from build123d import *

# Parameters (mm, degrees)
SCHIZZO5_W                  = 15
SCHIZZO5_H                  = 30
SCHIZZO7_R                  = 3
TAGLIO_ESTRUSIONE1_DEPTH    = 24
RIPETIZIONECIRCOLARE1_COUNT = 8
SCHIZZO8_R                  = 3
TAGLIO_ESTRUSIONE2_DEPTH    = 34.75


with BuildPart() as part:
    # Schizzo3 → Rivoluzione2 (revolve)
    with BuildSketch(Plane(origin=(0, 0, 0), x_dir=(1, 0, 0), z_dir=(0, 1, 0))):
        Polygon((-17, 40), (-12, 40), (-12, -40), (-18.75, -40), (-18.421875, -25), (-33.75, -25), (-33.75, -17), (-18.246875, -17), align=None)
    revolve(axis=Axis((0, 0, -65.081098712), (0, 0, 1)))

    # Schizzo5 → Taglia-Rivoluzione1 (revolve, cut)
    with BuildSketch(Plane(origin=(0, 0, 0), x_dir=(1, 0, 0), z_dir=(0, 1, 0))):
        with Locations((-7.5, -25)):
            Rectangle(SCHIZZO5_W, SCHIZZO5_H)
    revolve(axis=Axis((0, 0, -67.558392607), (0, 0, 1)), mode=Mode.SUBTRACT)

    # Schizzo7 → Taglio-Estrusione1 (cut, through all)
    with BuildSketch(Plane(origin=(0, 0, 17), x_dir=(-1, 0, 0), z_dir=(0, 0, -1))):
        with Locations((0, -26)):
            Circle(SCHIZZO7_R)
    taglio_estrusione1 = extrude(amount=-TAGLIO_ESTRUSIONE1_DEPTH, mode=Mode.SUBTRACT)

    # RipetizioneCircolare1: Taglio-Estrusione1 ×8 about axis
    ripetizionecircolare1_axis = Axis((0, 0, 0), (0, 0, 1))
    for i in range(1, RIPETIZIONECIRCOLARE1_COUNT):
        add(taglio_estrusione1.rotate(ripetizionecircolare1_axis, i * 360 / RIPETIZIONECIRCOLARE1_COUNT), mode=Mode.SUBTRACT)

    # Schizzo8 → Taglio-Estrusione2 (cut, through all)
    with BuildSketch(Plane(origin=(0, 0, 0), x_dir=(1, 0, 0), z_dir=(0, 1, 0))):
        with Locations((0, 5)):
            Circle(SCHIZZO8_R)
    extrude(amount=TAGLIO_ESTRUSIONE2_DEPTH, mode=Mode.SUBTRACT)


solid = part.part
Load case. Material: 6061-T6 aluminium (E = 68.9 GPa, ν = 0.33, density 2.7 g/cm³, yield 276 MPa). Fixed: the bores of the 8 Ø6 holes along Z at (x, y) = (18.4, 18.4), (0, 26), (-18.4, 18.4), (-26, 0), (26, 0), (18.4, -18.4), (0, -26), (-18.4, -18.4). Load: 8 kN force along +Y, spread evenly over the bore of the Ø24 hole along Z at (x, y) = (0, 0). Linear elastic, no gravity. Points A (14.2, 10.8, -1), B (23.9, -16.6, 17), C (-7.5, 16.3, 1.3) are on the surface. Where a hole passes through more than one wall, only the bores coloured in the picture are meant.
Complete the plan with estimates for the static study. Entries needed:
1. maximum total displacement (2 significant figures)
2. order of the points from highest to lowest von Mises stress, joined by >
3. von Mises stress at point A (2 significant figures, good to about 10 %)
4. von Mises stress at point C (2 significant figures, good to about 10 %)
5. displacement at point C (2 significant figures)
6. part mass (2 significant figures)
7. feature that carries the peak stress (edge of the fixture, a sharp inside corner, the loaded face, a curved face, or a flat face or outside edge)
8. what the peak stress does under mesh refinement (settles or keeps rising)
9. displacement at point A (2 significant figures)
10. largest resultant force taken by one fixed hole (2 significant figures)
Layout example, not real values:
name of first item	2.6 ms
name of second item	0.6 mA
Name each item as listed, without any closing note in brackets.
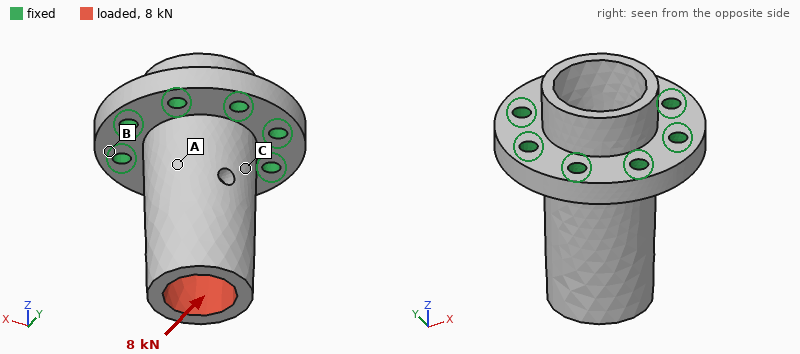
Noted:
maximum total displacement	0.14 mm
order of the points from highest to lowest von Mises stress, joined by >	C > A > B
von Mises stress at point A	30 MPa
von Mises stress at point C	42 MPa
displacement at point C	0.050 mm
part mass	150 g
feature that carries the peak stress	edge of the fixture
what the peak stress does under mesh refinement	keeps rising
displacement at point A	0.050 mm
largest resultant force taken by one fixed hole	3.7 kN
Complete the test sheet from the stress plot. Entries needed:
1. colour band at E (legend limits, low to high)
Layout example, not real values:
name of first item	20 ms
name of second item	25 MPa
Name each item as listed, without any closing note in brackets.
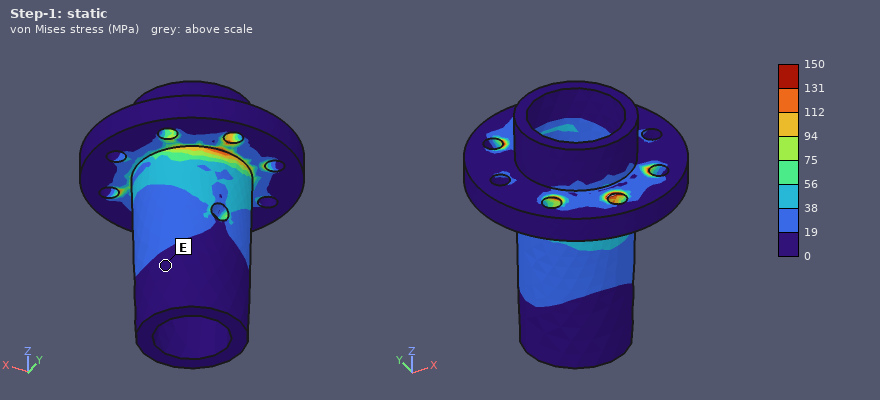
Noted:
colour band at E	0 to 19 MPa
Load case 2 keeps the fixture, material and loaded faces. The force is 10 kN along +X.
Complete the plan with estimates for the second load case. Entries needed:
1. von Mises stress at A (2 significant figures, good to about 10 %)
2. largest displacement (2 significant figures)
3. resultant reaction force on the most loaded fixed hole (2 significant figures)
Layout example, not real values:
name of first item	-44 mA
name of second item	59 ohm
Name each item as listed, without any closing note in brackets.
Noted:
von Mises stress at A	47 MPa
largest displacement	0.18 mm
resultant reaction force on the most loaded fixed hole	4.6 kN
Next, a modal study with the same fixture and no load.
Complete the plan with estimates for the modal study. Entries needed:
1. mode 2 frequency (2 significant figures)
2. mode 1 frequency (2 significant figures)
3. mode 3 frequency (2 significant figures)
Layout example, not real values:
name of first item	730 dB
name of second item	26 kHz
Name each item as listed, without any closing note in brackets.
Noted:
mode 2 frequency	5500 Hz
mode 1 frequency	5500 Hz
mode 3 frequency	13 kHz
